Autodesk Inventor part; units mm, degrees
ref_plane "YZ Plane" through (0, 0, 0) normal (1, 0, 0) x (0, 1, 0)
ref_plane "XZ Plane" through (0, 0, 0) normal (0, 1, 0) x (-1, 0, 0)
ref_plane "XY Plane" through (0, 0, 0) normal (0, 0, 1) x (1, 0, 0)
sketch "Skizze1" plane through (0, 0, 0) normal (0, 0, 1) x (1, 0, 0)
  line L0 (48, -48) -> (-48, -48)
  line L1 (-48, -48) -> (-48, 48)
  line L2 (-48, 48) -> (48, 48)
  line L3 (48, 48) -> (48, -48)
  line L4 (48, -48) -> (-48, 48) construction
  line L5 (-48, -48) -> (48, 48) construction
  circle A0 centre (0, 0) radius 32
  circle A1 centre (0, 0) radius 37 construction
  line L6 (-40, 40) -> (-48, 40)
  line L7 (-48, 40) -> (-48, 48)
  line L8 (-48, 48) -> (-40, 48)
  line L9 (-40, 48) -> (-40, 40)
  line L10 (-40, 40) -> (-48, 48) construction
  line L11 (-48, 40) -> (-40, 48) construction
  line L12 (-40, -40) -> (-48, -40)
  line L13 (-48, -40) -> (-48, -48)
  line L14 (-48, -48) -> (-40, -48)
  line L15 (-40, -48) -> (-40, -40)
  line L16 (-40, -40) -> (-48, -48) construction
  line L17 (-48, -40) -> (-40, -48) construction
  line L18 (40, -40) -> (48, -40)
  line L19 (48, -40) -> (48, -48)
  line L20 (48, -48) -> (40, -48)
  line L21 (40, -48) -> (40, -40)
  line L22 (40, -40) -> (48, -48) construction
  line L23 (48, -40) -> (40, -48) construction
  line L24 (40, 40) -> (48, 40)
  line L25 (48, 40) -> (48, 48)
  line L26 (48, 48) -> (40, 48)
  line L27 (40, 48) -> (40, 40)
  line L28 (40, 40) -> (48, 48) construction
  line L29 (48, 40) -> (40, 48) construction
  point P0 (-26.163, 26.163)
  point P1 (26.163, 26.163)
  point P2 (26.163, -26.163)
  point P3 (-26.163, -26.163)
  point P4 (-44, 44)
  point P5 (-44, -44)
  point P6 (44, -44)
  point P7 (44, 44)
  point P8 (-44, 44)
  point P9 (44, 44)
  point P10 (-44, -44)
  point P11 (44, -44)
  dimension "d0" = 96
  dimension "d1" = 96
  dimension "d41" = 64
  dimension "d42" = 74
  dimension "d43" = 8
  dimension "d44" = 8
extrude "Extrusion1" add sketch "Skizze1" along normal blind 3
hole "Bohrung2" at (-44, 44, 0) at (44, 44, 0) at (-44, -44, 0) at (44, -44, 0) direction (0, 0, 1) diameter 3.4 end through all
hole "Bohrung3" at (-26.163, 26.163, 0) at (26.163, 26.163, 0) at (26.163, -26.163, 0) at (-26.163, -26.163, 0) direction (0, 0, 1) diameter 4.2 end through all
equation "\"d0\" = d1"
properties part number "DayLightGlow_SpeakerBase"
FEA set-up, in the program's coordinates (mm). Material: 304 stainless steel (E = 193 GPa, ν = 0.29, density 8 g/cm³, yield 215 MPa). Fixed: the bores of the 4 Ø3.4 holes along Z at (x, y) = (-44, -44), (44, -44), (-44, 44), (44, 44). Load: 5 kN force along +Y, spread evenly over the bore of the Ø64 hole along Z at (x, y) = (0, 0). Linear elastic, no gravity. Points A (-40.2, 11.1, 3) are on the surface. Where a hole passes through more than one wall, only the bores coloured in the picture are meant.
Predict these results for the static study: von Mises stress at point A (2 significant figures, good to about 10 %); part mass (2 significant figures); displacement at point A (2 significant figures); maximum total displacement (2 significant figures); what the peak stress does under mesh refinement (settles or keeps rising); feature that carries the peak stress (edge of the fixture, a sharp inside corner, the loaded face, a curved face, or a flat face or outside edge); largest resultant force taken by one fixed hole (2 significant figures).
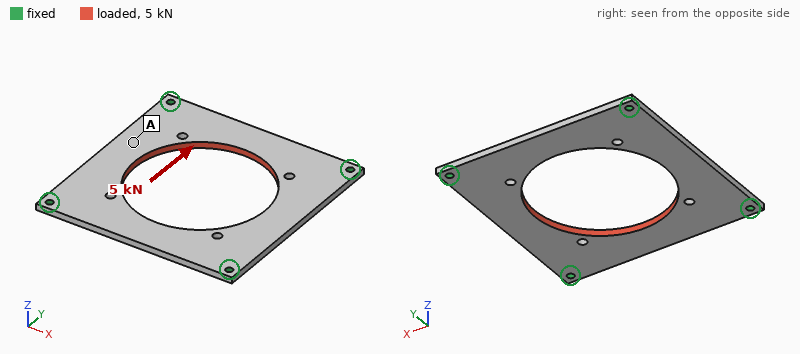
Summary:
20 MPa
140 g
5.4 µm
14 µm
keeps rising
edge of the fixture
1.4 kN
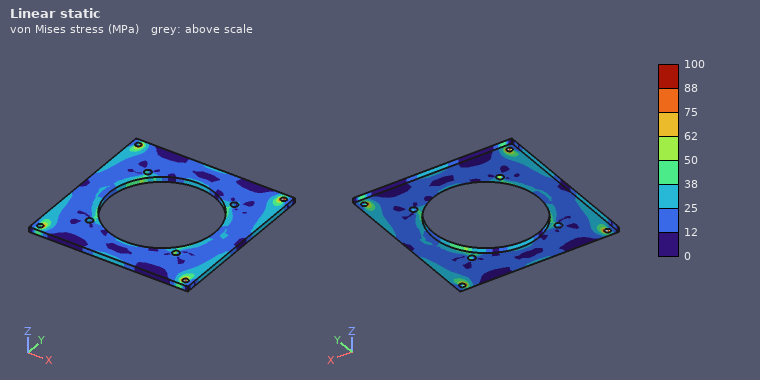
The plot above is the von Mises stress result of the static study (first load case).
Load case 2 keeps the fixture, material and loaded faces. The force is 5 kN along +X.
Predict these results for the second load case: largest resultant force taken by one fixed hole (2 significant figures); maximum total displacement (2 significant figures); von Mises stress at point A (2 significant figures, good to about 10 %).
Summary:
1.4 kN
14 µm
15 MPa
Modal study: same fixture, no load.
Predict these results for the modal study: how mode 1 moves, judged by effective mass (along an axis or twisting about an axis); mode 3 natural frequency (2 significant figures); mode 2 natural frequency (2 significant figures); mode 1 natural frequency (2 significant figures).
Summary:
along Z
2000 Hz
2000 Hz
1600 Hz
